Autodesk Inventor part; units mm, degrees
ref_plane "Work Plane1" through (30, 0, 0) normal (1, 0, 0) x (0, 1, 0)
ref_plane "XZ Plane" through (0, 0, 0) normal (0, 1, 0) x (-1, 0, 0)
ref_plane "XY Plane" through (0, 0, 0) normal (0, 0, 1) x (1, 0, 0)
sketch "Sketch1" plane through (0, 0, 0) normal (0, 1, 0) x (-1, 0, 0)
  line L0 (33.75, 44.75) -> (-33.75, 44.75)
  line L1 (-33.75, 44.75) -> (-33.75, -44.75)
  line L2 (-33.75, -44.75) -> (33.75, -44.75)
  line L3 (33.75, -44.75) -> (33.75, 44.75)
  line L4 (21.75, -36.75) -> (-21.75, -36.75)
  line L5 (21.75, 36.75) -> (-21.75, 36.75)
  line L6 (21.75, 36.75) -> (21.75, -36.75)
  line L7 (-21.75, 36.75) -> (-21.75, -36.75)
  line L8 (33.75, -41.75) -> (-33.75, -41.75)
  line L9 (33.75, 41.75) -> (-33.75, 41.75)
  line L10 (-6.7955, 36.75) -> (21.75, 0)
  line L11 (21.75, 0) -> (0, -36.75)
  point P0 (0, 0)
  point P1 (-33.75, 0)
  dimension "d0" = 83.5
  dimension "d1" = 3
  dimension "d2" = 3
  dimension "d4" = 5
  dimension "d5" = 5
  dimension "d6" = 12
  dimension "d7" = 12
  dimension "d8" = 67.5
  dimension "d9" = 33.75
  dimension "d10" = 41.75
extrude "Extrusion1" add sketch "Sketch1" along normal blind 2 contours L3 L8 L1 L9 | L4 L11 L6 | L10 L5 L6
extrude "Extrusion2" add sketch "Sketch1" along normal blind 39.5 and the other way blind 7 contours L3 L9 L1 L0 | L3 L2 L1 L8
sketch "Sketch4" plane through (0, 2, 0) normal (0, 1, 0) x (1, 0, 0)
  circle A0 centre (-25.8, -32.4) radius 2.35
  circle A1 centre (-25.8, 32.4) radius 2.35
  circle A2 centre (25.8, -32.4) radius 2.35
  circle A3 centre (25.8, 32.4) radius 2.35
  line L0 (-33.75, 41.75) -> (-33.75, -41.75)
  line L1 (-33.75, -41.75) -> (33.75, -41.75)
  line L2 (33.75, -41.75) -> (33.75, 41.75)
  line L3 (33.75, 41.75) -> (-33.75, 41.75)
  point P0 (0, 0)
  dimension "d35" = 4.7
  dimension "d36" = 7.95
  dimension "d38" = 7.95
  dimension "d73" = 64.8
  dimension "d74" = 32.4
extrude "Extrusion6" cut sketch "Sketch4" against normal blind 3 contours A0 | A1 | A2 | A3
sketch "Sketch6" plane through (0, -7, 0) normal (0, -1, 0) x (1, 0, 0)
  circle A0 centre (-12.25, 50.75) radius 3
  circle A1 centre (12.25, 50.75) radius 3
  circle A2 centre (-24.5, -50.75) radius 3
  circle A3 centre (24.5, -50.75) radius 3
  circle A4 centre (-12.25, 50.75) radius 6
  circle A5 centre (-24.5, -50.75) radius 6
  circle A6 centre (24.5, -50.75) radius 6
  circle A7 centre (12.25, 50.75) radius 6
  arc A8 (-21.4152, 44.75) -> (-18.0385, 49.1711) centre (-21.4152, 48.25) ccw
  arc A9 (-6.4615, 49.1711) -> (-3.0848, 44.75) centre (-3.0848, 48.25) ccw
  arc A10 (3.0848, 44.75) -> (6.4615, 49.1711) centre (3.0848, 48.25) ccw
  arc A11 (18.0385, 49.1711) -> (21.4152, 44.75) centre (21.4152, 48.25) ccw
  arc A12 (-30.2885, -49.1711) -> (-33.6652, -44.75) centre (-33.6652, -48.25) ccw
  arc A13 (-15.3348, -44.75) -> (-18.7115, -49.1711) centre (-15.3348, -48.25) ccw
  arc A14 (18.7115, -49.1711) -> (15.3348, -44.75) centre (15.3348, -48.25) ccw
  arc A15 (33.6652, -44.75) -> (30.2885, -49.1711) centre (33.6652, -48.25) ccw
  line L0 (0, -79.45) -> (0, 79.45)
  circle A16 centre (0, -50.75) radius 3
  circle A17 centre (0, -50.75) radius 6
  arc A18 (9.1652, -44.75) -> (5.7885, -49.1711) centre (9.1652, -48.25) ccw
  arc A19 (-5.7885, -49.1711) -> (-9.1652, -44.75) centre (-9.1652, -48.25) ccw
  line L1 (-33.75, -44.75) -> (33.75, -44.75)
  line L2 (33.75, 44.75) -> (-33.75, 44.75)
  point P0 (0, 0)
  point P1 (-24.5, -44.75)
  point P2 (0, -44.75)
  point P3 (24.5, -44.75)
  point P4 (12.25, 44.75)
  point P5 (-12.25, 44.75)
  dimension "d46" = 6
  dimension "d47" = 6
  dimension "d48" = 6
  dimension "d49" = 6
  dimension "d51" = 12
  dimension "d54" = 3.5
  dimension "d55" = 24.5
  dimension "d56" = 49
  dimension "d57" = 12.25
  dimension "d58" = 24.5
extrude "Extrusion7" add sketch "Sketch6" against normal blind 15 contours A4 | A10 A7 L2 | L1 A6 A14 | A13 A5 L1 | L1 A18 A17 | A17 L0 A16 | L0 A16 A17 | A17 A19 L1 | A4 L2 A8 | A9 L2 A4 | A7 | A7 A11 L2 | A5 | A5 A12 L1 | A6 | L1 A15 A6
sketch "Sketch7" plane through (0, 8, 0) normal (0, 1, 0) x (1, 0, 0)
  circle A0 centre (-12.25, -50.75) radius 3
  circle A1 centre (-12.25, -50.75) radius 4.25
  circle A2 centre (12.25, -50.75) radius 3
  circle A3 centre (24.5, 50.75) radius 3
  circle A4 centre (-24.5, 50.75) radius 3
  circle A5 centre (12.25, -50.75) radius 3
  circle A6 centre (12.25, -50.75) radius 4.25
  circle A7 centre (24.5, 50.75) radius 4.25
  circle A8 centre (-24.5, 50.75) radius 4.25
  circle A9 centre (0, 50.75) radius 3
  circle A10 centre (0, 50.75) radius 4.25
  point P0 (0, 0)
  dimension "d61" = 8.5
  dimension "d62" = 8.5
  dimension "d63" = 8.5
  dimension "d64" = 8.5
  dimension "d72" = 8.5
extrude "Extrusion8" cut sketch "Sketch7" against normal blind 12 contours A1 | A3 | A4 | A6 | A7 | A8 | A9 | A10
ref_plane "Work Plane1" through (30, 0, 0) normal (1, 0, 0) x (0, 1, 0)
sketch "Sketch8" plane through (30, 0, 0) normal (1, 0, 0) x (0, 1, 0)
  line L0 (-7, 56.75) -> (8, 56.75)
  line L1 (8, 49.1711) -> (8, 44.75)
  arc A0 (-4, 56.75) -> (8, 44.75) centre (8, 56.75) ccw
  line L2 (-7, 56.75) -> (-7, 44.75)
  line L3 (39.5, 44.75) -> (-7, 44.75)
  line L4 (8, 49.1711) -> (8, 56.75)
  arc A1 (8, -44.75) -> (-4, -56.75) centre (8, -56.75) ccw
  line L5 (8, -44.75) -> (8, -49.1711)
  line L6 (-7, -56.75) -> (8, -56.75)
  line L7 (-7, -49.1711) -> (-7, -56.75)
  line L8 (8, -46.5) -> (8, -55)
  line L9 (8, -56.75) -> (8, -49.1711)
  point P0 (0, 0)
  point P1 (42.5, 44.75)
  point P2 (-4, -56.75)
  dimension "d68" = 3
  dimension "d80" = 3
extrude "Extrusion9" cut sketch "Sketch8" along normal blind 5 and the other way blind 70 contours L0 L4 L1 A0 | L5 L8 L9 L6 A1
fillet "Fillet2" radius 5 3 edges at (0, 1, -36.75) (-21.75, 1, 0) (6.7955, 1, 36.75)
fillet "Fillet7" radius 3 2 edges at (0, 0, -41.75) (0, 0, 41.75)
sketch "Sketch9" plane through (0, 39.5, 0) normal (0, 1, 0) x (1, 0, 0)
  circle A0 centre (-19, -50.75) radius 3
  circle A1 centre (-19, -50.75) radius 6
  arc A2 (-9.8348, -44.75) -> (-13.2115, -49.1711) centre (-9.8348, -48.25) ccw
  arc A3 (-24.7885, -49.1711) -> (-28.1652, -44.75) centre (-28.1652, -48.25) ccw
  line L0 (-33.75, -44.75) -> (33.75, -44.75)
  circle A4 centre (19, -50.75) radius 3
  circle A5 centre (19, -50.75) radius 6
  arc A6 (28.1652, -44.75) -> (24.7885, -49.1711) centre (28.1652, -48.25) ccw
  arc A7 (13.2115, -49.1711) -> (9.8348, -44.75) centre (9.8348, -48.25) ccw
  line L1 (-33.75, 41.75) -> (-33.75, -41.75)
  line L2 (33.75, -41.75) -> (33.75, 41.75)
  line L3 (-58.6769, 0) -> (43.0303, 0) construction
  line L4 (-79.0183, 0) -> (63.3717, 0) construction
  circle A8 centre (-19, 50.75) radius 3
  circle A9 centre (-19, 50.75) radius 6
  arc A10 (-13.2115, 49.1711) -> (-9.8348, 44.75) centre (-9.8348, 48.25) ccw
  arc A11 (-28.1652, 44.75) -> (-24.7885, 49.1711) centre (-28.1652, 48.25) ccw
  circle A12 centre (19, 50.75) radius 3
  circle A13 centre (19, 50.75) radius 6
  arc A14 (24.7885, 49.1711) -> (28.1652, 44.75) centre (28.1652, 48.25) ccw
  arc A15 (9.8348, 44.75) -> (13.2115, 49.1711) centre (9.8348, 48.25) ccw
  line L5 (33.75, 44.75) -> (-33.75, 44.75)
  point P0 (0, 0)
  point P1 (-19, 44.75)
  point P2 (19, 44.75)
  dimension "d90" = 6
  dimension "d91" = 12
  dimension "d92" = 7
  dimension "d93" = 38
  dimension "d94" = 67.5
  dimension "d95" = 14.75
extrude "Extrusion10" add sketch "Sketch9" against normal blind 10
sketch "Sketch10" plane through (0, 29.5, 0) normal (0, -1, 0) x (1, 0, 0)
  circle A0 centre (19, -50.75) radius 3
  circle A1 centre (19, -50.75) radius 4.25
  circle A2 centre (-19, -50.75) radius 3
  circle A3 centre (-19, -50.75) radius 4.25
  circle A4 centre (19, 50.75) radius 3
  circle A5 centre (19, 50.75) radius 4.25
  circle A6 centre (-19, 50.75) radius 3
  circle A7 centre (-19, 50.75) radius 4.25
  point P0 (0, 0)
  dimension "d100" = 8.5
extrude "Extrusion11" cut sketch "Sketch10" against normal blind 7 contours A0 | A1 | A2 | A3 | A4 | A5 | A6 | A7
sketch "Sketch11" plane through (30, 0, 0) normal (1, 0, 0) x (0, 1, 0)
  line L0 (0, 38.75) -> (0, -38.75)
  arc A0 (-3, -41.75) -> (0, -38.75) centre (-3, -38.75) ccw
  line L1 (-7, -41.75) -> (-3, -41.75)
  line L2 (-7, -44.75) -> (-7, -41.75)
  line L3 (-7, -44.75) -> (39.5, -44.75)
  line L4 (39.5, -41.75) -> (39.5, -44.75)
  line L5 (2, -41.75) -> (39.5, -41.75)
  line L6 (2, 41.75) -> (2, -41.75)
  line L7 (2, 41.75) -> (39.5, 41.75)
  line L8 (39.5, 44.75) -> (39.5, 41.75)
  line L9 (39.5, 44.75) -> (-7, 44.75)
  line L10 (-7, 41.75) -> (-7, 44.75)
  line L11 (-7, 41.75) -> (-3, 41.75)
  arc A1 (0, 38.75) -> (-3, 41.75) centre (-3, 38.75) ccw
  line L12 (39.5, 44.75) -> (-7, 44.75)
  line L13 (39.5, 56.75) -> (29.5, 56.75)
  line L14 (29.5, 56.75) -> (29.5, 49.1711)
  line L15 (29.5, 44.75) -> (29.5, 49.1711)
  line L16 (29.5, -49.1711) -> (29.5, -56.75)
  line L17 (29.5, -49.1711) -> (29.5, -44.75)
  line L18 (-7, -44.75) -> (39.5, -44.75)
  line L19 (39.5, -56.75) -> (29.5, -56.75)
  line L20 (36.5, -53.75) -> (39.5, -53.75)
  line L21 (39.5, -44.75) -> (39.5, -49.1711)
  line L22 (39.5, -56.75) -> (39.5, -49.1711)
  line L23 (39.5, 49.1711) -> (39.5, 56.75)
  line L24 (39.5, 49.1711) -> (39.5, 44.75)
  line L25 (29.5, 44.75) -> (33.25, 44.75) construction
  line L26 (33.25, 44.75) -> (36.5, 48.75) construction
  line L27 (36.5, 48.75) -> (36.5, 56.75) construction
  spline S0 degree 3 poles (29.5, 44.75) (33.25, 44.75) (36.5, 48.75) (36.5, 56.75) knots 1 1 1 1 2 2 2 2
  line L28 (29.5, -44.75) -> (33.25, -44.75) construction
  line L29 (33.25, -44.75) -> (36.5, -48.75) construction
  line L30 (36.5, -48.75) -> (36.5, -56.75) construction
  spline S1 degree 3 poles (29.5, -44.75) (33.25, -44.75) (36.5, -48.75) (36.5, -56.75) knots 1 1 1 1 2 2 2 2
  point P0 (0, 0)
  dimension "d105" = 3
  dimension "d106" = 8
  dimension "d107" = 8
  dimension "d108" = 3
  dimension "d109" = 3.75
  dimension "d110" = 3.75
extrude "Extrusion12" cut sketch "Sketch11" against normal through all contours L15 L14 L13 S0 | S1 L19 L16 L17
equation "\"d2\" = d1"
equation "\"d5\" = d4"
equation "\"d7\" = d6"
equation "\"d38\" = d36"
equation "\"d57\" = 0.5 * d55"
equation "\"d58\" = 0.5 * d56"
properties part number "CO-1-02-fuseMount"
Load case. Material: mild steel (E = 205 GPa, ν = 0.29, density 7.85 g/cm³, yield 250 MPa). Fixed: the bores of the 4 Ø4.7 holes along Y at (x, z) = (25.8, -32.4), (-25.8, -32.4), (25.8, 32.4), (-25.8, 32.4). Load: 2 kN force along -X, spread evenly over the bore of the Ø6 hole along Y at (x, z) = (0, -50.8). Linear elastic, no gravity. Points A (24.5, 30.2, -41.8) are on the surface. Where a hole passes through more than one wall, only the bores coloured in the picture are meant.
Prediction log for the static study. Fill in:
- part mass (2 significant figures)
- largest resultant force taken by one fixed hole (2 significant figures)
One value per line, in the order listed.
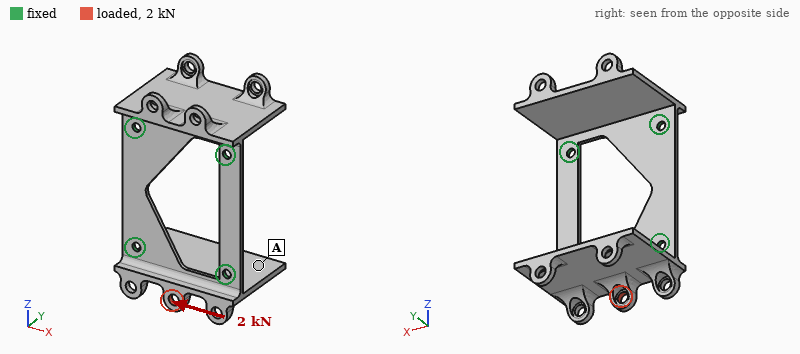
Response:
240 g
1.3 kN
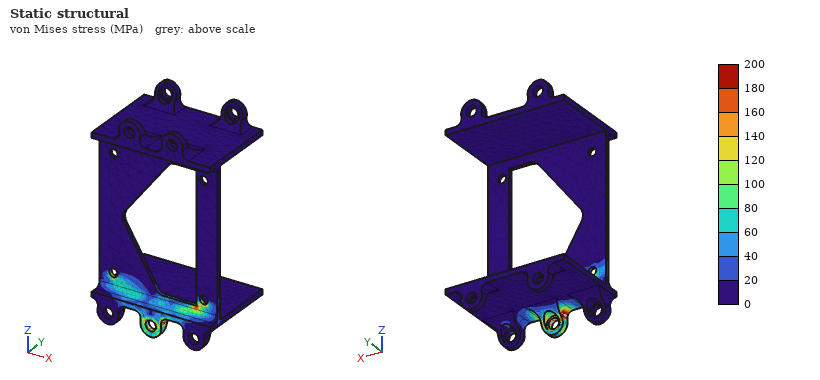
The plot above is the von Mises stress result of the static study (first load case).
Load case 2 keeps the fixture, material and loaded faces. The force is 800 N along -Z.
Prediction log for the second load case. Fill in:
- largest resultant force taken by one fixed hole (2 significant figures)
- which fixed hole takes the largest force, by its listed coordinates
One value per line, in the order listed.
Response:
570 N
(-25.8, -32.4)
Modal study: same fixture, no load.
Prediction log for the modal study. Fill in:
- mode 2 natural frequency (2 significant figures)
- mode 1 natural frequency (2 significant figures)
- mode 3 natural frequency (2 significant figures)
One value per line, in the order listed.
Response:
600 Hz
590 Hz
2100 Hz
